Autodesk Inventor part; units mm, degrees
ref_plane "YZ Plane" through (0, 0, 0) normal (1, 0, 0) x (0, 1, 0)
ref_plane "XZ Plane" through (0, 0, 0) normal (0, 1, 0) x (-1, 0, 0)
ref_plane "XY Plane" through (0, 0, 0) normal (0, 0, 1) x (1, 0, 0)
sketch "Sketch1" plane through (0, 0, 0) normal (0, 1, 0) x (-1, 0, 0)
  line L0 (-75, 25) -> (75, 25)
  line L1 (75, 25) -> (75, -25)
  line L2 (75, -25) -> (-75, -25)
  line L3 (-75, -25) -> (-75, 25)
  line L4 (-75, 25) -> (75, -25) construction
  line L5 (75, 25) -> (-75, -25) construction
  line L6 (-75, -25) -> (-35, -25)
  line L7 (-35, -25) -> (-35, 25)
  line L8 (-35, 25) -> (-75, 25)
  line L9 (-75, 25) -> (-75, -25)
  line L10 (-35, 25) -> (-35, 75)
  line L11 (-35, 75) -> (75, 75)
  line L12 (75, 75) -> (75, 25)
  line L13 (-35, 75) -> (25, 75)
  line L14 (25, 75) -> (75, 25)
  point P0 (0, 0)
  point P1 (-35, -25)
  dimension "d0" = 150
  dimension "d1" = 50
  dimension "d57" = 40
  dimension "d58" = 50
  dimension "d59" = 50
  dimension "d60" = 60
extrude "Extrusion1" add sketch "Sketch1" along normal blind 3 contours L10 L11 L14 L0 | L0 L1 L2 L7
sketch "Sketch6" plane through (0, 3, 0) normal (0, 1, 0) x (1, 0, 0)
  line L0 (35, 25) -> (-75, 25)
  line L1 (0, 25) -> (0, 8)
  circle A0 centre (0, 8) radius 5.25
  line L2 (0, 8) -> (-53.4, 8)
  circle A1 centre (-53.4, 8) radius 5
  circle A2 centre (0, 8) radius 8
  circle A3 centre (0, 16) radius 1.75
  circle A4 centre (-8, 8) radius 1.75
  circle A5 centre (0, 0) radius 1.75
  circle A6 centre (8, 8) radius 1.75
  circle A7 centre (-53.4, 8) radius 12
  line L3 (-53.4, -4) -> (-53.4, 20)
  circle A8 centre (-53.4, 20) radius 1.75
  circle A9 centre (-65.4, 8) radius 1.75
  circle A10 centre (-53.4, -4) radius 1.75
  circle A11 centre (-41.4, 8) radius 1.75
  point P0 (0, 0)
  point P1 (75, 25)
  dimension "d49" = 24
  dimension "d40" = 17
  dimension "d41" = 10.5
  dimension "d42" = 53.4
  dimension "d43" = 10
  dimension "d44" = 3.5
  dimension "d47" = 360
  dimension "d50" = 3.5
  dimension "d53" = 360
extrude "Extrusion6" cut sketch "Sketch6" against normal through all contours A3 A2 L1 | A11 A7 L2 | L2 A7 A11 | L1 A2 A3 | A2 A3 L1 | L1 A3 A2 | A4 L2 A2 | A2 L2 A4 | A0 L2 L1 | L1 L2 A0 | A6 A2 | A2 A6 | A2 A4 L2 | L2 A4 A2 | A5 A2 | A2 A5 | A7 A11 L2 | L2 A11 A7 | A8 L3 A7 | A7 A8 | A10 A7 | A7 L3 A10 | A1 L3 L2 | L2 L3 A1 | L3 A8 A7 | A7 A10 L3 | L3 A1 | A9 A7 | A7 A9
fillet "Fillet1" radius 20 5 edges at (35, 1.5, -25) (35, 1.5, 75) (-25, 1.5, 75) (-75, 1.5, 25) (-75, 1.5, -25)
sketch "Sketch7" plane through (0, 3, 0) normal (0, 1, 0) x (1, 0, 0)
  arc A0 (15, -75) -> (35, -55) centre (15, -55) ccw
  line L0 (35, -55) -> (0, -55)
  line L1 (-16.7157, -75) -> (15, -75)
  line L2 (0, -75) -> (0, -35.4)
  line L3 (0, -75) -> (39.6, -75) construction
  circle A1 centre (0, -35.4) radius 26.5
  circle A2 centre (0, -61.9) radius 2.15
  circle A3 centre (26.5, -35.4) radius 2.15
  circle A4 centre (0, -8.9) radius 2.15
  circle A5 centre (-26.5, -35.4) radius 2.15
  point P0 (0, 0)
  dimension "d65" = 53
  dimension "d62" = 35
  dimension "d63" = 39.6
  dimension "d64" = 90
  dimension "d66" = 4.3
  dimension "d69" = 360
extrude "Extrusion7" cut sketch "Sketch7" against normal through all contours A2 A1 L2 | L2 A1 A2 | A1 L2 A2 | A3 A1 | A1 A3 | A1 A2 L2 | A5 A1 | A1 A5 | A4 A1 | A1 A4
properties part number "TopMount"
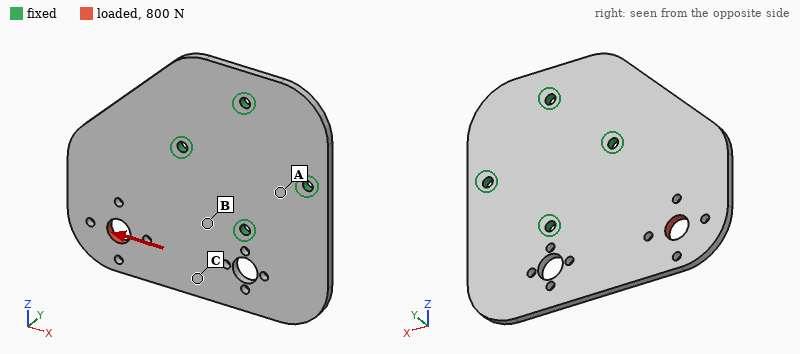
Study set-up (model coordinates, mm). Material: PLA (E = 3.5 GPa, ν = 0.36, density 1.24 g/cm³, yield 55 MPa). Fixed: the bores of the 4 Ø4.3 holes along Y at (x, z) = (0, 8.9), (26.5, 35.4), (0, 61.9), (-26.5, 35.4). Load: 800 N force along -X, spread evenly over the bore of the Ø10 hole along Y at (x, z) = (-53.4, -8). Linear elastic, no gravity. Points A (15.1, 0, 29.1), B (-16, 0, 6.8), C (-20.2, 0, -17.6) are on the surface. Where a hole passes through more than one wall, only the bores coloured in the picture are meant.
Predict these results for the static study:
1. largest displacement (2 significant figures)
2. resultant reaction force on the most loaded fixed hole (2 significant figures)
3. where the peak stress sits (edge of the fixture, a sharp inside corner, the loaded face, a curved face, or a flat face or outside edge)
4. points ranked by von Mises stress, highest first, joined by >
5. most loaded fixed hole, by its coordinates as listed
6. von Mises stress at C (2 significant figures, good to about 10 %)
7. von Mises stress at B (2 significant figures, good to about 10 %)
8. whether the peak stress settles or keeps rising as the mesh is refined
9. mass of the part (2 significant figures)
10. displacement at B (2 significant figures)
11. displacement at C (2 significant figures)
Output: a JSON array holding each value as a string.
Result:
["0.27 mm", "710 N", "edge of the fixture", "B > C > A", "(0, 8.9)", "5.0 MPa", "9.2 MPa", "keeps rising", "34 g", "0.055 mm", "0.15 mm"]
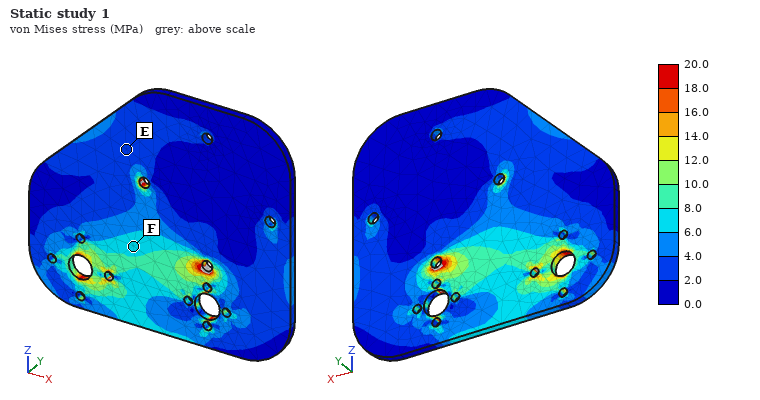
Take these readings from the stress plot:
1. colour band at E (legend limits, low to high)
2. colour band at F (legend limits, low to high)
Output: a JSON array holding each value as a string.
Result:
["2.0 to 4.0 MPa", "6.0 to 8.0 MPa"]
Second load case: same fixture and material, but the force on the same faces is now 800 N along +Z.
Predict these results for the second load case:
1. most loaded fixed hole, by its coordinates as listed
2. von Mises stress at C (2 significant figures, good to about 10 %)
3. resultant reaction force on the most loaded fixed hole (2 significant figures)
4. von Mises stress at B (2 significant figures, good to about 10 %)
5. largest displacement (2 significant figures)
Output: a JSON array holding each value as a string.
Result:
["(-26.5, 35.4)", "3.1 MPa", "770 N", "5.2 MPa", "0.30 mm"]
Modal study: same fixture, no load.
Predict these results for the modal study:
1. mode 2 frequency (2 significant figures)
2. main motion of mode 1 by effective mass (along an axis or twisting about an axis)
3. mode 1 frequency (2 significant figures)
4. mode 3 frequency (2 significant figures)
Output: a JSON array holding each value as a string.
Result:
["530 Hz", "along Y", "240 Hz", "640 Hz"]
